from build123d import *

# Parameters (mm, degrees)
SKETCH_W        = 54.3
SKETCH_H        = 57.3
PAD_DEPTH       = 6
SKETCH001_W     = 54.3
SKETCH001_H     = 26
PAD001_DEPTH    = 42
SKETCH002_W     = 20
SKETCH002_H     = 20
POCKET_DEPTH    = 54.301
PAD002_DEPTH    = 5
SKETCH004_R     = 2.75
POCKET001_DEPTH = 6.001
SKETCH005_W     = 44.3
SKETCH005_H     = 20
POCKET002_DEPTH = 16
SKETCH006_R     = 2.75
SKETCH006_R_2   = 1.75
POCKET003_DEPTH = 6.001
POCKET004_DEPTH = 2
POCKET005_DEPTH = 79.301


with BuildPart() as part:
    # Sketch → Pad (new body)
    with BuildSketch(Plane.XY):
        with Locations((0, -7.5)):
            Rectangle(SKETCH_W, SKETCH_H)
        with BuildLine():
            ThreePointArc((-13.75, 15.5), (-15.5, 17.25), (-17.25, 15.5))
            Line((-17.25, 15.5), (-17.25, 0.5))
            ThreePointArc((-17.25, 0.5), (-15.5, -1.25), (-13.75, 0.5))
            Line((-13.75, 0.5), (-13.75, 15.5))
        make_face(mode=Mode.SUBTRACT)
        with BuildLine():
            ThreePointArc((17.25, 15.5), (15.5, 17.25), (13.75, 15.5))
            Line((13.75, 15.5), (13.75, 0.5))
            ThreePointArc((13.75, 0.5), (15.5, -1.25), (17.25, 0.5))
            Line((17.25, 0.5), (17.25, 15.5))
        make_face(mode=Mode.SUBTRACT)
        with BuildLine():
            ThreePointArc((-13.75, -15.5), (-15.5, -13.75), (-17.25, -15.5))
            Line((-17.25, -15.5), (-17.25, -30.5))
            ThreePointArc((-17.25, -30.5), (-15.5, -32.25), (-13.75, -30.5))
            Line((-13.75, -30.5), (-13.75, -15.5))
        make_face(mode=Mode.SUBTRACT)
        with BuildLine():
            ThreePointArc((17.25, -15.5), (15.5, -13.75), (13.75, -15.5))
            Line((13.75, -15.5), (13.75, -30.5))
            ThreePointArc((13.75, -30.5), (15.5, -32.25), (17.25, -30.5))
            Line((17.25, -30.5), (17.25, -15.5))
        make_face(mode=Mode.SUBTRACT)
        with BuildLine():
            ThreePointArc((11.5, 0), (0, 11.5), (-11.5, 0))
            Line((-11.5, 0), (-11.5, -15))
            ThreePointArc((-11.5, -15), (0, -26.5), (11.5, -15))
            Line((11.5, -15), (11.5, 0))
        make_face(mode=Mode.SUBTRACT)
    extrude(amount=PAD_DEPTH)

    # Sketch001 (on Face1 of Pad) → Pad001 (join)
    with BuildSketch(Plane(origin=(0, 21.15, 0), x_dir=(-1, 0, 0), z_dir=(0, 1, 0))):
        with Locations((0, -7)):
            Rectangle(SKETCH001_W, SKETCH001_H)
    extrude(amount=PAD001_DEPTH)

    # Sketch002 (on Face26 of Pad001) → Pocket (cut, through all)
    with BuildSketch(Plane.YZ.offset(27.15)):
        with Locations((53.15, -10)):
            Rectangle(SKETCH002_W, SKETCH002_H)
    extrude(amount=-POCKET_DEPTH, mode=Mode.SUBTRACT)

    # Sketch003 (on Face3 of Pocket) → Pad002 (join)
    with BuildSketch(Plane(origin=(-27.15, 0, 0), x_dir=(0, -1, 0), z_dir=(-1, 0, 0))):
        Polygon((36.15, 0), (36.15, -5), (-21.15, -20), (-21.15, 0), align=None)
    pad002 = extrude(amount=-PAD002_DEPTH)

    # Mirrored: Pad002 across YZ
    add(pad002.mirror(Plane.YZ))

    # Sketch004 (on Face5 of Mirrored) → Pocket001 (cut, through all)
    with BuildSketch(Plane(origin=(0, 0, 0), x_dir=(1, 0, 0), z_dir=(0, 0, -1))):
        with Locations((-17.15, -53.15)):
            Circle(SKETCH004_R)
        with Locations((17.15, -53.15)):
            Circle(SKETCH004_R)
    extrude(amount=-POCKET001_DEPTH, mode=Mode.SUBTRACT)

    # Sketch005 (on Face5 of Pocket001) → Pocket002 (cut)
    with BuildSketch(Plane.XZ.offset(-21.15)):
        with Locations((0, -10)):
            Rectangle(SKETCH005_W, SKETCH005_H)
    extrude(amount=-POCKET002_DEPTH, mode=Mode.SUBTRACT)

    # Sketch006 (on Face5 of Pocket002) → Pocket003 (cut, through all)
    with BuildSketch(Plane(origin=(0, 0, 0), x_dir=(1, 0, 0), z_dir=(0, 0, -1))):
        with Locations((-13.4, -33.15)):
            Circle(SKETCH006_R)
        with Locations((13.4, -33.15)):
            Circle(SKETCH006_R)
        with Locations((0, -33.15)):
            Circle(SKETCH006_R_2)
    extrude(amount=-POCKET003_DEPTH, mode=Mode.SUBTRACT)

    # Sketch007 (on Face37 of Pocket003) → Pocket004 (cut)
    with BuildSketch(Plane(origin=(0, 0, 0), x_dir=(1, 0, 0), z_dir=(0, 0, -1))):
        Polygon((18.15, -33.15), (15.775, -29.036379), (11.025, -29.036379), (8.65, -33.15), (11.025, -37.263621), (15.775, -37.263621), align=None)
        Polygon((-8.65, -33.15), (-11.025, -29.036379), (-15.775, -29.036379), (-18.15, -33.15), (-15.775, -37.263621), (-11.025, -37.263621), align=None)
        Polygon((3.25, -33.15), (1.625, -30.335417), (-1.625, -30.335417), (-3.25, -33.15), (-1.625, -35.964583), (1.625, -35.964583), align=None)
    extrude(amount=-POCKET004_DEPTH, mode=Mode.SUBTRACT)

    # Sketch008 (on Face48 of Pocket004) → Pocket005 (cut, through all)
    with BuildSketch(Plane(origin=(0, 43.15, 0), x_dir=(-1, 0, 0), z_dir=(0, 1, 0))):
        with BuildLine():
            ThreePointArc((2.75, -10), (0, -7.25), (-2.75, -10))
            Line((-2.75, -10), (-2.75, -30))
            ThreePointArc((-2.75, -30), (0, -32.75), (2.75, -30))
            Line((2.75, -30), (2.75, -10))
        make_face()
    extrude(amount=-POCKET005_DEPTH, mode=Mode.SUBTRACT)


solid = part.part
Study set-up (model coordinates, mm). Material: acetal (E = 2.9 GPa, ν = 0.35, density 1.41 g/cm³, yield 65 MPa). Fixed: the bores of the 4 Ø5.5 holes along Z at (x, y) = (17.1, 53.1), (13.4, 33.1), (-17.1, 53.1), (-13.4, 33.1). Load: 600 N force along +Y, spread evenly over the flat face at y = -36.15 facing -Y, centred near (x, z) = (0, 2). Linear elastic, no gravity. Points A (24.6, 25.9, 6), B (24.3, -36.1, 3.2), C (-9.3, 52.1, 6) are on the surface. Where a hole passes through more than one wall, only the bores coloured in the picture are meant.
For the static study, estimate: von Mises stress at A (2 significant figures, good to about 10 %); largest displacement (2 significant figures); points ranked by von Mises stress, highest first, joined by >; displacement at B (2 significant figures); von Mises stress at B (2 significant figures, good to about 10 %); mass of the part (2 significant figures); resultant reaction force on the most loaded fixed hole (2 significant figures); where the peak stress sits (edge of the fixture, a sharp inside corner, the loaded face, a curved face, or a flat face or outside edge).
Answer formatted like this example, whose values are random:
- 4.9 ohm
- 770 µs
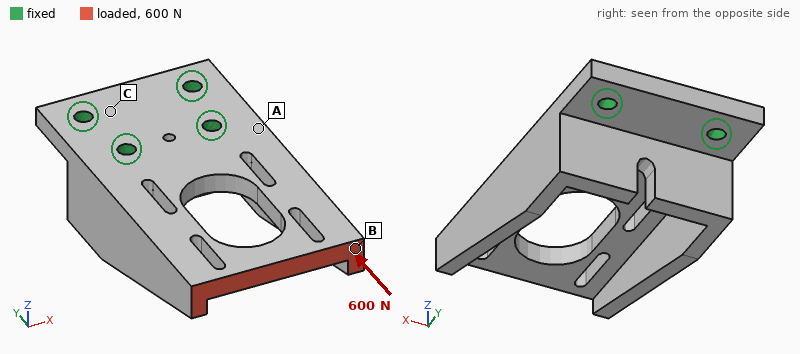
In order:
- 2.9 MPa
- 0.15 mm
- A > B > C
- 0.094 mm
- 1.8 MPa
- 59 g
- 200 N
- a curved face
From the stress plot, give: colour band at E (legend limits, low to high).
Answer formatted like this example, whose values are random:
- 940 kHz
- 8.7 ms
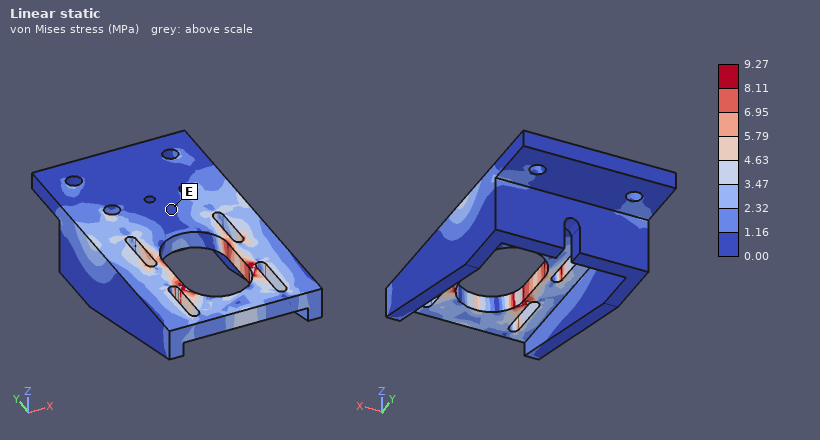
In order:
- 0.00 to 1.16 MPa
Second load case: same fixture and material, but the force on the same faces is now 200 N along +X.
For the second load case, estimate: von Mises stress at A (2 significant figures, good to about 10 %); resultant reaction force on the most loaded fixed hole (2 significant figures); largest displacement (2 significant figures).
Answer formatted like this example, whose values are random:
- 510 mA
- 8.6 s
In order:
- 4.8 MPa
- 250 N
- 0.60 mm
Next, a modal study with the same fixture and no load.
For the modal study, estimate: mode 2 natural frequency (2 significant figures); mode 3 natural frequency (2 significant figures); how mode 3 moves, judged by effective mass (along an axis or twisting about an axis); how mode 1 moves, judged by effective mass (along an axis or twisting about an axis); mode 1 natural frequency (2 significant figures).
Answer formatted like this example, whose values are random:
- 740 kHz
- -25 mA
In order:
- 730 Hz
- 1100 Hz
- along X
- along Z
- 570 Hz
